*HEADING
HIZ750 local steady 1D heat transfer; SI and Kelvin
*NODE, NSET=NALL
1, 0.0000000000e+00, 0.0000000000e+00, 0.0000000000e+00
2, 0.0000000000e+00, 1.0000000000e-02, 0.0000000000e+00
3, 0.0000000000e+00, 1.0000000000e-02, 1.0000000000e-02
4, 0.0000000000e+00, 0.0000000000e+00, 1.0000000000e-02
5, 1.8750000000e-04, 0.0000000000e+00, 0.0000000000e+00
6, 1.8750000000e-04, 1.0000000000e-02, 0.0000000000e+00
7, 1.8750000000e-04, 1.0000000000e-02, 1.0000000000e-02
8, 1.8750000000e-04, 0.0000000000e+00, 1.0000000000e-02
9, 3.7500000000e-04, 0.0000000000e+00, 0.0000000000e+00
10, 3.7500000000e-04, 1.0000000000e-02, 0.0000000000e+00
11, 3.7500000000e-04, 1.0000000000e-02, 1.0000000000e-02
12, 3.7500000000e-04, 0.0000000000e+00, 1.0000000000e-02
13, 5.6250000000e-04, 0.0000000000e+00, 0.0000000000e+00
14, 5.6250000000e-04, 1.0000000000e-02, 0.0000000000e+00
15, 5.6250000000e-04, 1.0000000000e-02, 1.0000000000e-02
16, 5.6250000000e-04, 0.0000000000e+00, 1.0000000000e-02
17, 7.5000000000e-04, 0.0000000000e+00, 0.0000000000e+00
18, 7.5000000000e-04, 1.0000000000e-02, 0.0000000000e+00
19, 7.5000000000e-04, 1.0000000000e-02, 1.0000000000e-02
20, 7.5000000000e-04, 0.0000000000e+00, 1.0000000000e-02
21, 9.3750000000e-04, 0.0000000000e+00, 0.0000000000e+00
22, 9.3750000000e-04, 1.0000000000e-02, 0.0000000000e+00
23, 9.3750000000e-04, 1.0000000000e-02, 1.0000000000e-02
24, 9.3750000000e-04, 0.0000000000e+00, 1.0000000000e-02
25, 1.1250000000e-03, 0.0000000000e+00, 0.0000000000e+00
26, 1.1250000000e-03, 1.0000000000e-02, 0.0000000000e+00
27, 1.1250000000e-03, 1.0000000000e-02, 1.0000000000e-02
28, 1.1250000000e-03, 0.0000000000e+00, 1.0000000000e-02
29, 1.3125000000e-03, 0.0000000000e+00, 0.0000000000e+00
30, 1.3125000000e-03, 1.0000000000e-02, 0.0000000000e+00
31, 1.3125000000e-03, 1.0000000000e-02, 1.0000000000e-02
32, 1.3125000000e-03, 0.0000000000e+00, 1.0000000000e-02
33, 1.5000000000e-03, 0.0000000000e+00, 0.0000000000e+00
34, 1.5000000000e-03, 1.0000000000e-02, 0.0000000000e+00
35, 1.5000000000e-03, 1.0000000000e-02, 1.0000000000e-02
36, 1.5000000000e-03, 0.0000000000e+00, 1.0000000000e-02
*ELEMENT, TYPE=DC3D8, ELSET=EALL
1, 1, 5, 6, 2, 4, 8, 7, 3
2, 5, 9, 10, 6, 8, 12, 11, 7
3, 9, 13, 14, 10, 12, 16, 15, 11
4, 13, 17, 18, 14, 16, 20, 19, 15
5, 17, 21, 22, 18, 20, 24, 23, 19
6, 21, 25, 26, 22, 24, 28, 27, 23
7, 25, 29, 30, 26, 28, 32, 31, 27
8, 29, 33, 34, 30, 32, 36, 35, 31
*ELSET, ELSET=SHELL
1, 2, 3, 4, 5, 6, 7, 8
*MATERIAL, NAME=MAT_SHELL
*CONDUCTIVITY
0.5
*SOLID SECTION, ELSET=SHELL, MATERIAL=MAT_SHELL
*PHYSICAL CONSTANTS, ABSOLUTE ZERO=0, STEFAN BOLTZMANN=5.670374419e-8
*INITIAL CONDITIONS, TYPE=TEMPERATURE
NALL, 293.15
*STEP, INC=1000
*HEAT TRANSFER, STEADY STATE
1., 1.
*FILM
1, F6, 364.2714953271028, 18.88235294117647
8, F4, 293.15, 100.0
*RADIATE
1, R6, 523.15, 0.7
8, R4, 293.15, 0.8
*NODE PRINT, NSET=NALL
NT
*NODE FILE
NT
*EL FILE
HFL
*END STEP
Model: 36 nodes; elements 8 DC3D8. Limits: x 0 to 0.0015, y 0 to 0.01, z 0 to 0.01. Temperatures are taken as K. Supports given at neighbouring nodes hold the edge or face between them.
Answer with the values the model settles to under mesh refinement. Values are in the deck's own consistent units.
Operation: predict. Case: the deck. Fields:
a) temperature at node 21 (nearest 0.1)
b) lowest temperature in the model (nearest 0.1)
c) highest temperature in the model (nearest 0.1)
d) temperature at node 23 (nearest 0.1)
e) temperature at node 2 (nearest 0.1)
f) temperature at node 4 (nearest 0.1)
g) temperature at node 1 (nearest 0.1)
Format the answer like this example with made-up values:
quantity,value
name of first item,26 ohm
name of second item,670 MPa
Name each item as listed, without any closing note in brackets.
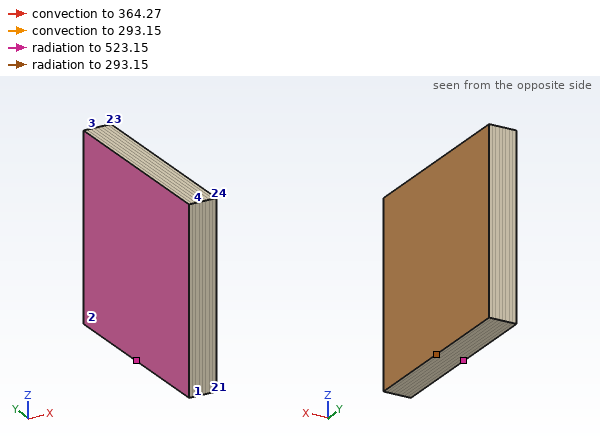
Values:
quantity,value
temperature at node 21,326.1 K
lowest temperature in the model,322.6 K
highest temperature in the model,331.9 K
temperature at node 23,326.1 K
temperature at node 2,331.9 K
temperature at node 4,331.9 K
temperature at node 1,331.9 K
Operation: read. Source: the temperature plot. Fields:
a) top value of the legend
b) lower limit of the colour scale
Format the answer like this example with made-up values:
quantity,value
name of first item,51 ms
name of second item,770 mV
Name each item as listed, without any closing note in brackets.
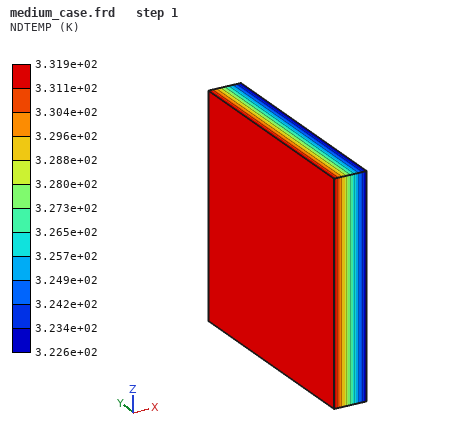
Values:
quantity,value
top value of the legend,3.319e+02 K
lower limit of the colour scale,3.226e+02 K
